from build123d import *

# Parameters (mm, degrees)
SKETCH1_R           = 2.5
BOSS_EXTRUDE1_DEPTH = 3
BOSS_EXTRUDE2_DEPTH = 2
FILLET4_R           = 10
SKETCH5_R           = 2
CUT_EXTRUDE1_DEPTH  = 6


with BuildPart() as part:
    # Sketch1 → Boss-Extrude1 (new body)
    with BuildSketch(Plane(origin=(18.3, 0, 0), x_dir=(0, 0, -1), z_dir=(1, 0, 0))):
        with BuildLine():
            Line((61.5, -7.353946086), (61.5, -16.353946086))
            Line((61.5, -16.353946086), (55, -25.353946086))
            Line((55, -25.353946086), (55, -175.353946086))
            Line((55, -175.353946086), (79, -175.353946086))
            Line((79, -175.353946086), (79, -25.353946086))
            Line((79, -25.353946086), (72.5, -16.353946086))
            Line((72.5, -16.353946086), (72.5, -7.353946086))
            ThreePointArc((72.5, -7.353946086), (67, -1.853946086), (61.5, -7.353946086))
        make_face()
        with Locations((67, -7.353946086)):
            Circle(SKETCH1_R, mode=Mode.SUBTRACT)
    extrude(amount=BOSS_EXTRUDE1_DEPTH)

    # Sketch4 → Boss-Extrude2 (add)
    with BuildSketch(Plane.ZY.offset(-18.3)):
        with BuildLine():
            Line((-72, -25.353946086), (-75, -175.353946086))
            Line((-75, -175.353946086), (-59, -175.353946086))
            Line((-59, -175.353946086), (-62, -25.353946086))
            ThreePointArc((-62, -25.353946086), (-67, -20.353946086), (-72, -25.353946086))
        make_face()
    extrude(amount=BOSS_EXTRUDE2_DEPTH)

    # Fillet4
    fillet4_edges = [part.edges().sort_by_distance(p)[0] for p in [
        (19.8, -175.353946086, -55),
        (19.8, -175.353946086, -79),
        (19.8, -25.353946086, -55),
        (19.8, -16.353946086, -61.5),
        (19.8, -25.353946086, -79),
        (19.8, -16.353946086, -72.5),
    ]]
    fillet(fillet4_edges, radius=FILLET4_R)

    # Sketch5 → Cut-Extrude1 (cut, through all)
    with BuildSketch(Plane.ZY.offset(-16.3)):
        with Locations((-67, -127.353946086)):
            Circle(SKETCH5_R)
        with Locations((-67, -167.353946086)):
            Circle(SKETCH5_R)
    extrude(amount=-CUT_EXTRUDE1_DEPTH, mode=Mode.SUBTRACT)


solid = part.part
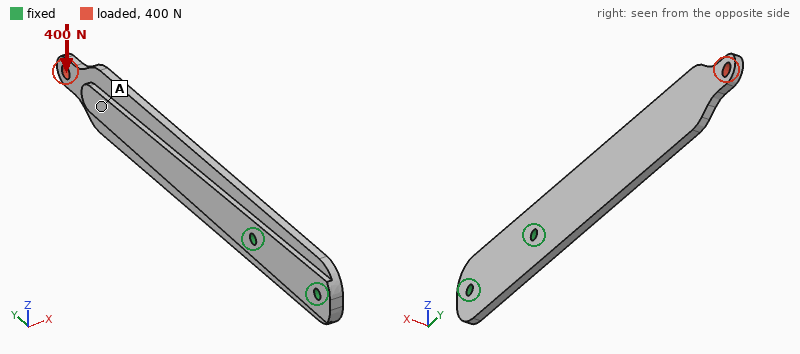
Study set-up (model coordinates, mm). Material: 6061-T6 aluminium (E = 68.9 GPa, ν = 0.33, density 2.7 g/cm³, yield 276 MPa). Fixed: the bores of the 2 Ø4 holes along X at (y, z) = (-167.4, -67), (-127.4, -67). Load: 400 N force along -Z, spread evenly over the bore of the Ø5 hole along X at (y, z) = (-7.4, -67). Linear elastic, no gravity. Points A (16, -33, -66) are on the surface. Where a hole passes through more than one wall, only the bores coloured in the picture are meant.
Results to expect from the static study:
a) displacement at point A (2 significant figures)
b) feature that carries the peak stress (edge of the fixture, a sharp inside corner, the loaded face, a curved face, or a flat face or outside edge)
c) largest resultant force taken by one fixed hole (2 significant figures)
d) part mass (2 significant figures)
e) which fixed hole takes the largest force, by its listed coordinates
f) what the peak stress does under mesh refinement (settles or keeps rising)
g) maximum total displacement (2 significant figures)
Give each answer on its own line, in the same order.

0.80 mm
edge of the fixture
1.3 kN
41 g
(-127.4, -67)
keeps rising
1.2 mm
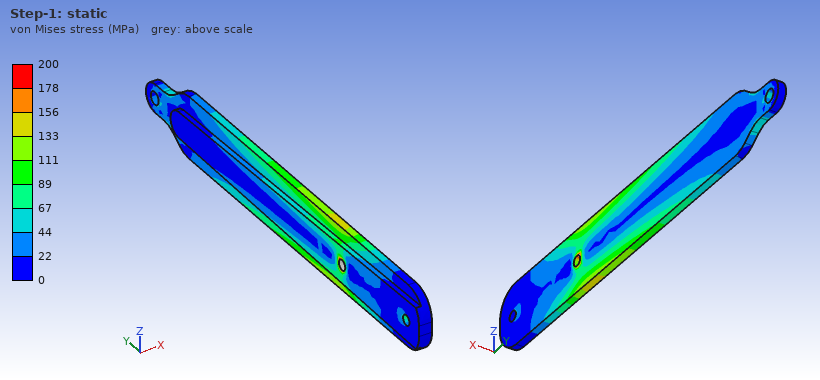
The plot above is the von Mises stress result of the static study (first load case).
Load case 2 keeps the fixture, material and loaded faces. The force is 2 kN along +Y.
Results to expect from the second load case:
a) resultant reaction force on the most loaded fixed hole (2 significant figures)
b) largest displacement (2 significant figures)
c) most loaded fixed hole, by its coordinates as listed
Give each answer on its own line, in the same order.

1.8 kN
0.84 mm
(-127.4, -67)
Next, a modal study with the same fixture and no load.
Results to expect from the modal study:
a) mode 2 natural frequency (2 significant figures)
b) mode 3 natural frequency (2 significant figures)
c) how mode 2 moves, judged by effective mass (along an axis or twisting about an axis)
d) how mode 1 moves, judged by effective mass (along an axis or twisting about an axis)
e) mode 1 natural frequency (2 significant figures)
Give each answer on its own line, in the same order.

1200 Hz
1800 Hz
along Z
along X
310 Hz
